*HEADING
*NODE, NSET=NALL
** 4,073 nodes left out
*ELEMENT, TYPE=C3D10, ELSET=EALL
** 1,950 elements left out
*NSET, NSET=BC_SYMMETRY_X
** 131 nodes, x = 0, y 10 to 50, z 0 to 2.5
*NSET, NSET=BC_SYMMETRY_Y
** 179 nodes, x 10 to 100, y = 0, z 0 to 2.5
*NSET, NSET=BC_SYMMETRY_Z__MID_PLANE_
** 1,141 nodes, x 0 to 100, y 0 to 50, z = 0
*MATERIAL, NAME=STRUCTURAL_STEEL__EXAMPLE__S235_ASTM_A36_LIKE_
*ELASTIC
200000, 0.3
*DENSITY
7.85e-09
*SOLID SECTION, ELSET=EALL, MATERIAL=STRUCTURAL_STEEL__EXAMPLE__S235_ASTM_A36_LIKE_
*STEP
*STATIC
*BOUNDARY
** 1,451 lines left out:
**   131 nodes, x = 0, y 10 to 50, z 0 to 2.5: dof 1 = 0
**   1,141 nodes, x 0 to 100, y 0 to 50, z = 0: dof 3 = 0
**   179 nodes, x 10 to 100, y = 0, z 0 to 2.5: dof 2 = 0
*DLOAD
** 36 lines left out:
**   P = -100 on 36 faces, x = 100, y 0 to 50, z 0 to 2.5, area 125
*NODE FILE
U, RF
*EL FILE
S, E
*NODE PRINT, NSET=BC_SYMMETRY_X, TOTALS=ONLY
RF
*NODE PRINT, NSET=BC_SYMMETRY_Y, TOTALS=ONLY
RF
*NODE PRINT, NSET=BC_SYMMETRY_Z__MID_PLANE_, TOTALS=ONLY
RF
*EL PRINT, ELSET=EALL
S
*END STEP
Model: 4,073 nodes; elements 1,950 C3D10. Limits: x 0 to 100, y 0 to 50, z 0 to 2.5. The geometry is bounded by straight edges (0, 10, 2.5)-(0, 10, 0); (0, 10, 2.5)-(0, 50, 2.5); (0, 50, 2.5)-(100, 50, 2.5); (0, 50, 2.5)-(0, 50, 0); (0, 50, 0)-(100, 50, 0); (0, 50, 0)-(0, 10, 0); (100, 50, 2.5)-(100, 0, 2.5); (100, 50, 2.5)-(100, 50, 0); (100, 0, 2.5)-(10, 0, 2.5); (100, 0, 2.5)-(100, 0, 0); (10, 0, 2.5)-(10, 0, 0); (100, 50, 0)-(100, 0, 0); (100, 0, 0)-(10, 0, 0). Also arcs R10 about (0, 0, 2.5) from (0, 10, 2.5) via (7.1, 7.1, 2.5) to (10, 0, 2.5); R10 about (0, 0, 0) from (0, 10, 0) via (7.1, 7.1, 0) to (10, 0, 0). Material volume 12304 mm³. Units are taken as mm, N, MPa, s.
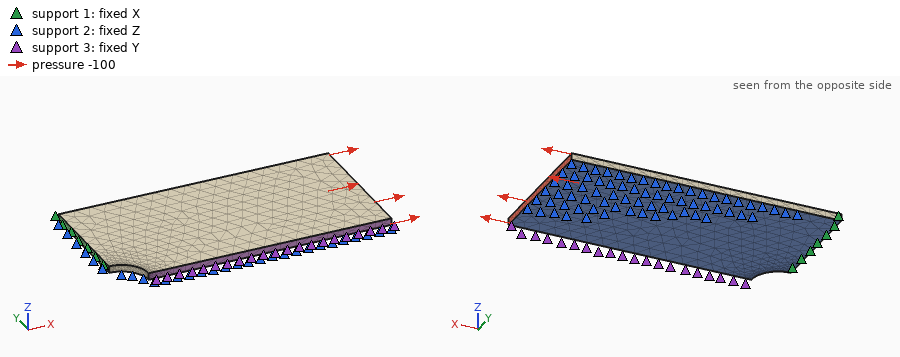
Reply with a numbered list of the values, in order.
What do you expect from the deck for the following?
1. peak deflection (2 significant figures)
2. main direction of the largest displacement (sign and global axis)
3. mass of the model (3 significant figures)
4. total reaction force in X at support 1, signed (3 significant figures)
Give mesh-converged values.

1. 0.053 mm
2. +X
3. 0.0966 kg
4. -12500 N
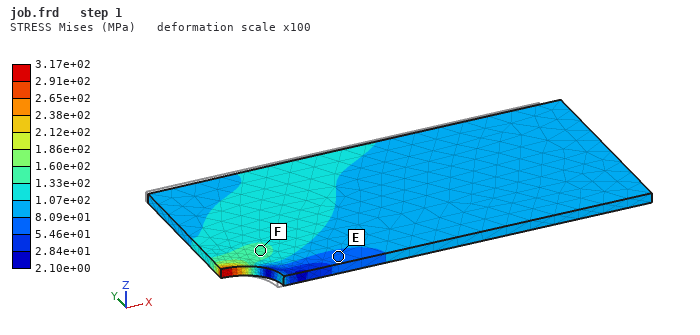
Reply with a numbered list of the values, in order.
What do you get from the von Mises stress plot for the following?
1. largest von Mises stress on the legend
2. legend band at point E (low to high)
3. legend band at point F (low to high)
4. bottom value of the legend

1. 3.17e+02 MPa
2. 5.46e+01 to 8.09e+01 MPa
3. 1.33e+02 to 1.60e+02 MPa
4. 2.10e+00 MPa
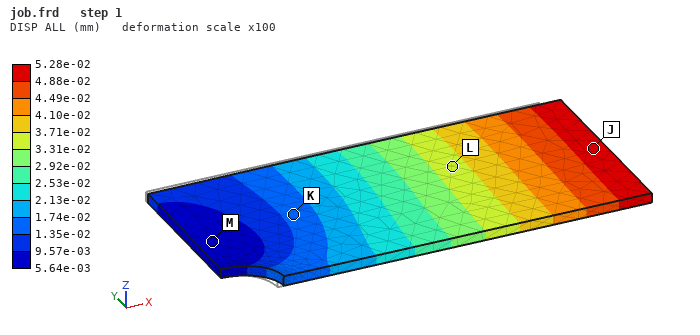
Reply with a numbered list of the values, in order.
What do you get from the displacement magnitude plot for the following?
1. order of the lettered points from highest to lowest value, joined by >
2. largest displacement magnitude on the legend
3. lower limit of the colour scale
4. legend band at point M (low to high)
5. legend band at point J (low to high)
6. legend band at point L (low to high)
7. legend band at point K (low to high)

1. J > L > K > M
2. 5.28e-02 mm
3. 5.64e-03 mm
4. 5.64e-03 to 9.57e-03 mm
5. 4.88e-02 to 5.28e-02 mm
6. 3.31e-02 to 3.71e-02 mm
7. 1.35e-02 to 1.74e-02 mm
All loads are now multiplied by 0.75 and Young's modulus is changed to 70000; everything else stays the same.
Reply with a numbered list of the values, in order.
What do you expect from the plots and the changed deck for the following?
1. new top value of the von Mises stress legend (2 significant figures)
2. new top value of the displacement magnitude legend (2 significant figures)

1. 240 MPa
2. 0.11 mm
